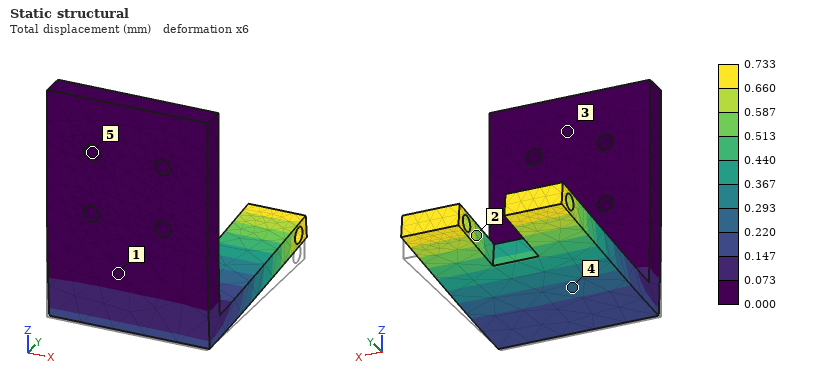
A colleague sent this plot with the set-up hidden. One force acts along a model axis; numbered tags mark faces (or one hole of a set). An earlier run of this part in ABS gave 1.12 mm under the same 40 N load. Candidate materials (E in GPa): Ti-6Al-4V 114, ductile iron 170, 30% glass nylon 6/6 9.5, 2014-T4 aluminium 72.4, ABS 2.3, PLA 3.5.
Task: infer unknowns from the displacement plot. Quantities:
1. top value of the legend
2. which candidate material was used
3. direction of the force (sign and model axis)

0.733 mm
PLA
+Z
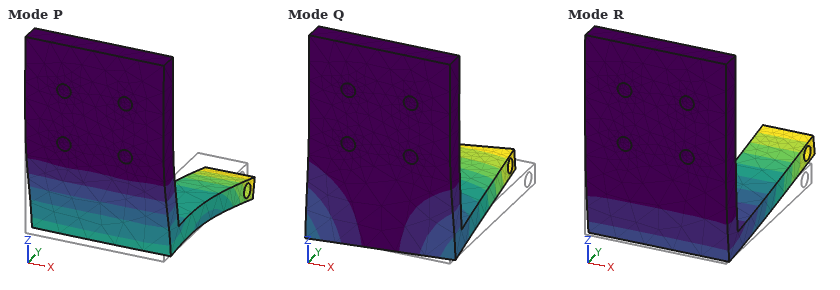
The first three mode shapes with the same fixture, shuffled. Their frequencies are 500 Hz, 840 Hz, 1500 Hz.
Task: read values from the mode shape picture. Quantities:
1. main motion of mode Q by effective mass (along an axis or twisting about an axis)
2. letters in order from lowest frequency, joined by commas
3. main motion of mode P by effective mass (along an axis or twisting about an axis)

along X
R, Q, P
along Y
